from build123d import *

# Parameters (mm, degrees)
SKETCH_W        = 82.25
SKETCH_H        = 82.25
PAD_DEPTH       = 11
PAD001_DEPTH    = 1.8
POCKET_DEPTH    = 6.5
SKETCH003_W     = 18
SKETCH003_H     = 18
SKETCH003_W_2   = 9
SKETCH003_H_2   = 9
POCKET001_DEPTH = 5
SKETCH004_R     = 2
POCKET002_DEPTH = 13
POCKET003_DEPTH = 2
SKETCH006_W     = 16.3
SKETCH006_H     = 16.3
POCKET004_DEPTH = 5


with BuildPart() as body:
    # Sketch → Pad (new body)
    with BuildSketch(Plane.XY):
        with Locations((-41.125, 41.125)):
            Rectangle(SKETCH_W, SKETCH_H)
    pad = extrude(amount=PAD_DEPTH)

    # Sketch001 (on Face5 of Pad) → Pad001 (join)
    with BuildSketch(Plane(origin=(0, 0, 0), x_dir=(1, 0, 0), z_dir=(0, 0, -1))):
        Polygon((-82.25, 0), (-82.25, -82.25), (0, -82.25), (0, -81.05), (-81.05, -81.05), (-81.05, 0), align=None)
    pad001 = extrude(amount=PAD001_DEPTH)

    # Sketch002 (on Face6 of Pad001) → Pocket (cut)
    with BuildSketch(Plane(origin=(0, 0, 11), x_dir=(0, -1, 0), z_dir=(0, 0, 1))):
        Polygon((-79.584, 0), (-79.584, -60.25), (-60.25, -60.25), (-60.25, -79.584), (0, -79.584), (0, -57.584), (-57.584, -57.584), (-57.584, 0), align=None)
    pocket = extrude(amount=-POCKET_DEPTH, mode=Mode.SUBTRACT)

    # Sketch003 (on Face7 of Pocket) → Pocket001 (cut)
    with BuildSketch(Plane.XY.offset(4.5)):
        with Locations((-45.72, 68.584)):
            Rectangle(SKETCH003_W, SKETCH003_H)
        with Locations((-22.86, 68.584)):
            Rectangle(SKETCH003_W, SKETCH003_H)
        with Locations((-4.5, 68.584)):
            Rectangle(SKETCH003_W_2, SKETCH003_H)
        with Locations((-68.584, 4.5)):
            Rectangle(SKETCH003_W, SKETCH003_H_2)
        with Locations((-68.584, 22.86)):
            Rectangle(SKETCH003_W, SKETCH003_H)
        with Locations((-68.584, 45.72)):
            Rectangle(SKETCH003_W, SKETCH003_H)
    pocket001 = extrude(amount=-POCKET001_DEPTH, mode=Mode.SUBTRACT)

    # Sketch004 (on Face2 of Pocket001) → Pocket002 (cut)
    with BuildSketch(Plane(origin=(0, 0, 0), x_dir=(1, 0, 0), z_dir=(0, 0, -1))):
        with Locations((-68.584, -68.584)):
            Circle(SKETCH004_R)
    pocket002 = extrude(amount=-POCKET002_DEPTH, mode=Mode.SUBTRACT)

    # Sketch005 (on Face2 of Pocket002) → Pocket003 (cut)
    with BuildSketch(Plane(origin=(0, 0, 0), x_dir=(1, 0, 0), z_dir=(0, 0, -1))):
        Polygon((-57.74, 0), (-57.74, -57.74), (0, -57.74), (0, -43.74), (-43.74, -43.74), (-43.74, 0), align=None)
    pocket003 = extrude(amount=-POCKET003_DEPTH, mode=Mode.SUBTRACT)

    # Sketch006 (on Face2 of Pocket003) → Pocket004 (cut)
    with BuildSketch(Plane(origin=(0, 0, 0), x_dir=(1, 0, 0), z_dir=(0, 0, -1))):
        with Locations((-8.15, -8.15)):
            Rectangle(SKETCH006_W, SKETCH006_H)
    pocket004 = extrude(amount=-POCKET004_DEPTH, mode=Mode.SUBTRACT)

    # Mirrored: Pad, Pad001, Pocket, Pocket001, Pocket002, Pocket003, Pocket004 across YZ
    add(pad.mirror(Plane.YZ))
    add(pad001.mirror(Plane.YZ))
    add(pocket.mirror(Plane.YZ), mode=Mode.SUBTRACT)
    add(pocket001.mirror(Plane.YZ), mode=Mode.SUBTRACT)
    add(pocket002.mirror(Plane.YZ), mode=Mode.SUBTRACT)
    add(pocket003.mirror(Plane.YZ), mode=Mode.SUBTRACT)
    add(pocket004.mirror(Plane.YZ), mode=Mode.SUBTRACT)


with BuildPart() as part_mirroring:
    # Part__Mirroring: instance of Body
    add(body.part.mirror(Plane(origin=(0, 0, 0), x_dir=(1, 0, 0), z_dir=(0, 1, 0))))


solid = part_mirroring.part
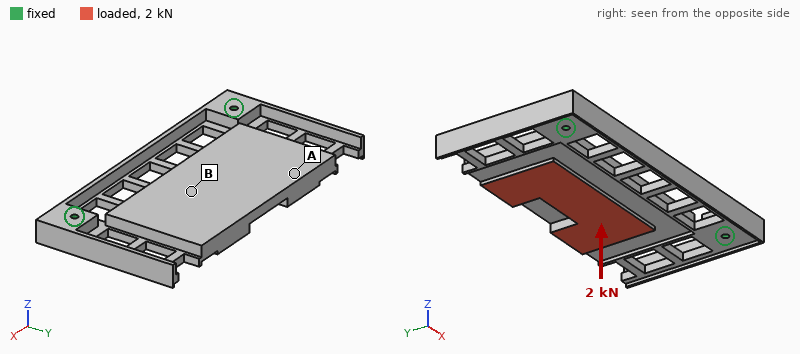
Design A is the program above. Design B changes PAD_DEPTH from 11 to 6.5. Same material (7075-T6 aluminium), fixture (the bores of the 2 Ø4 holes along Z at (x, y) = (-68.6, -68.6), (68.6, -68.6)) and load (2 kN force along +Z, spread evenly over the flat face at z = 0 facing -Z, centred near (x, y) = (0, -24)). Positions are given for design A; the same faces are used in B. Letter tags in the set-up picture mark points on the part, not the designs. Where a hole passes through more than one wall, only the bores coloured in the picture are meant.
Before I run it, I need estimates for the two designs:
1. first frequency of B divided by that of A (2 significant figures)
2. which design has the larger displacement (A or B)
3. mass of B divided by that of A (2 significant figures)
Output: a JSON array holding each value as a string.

["0.90", "B", "0.60"]
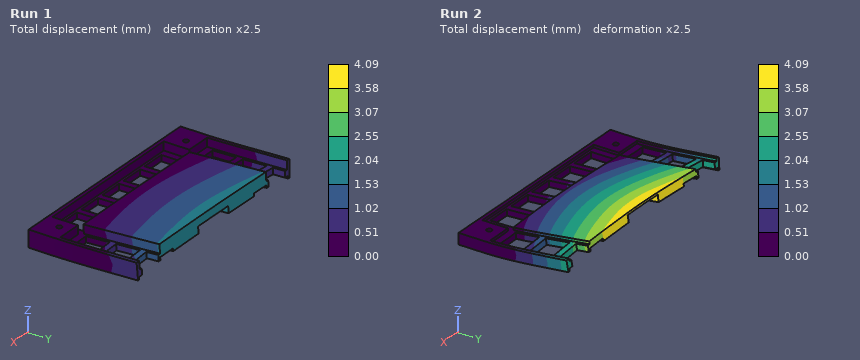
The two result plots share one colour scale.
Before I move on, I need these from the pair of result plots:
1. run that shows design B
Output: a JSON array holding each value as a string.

["Run 2"]
